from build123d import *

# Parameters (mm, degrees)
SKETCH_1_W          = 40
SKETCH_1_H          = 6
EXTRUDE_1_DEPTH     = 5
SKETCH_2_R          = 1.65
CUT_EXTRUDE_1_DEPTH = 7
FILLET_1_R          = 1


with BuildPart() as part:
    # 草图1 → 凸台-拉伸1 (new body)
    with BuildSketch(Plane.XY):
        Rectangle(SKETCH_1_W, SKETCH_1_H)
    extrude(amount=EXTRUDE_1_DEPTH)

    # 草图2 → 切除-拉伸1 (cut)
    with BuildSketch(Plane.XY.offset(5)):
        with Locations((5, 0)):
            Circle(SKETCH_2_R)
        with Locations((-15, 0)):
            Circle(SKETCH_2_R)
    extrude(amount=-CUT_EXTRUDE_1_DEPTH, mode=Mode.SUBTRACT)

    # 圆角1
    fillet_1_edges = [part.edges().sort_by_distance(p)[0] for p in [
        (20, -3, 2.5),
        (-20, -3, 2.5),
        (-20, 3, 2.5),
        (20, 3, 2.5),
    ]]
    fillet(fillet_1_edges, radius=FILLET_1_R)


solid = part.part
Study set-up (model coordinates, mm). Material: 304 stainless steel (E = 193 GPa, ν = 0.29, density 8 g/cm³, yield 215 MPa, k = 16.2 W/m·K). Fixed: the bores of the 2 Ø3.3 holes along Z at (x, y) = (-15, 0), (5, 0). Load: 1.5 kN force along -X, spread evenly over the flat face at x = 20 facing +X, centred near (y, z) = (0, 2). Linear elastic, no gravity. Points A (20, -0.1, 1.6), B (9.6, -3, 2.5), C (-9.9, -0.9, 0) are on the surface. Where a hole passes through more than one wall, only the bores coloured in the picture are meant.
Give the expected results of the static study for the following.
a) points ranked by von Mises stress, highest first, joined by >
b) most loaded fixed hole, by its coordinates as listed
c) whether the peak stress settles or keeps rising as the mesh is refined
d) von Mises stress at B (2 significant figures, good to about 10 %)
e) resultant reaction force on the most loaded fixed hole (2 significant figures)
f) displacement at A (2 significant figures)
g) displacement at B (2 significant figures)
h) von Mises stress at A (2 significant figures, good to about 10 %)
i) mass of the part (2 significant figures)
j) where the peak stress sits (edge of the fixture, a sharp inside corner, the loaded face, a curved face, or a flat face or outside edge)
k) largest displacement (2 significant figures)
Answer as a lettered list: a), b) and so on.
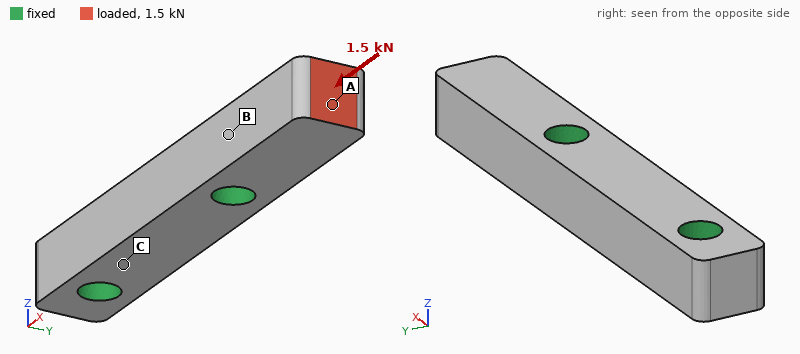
a) A > B > C
b) (5, 0)
c) keeps rising
d) 46 MPa
e) 1.5 kN
f) 4.0 µm
g) 1.0 µm
h) 61 MPa
i) 8.9 g
j) edge of the fixture
k) 4.1 µm
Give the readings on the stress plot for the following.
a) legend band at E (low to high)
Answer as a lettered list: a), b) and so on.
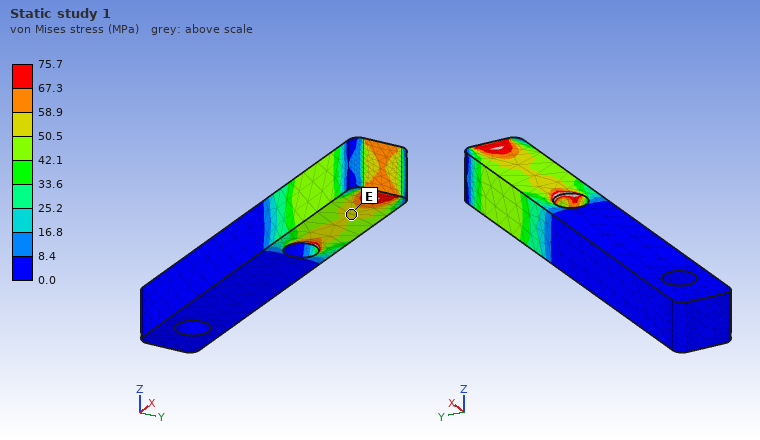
a) 50.5 to 58.9 MPa
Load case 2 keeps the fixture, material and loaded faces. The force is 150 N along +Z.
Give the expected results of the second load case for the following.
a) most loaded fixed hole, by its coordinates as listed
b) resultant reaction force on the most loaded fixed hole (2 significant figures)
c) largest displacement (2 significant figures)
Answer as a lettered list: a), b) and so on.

a) (5, 0)
b) 150 N
c) 13 µm
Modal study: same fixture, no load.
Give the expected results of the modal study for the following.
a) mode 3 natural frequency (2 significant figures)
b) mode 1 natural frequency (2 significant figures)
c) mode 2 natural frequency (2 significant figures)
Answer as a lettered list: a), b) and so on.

a) 50 kHz
b) 19 kHz
c) 19 kHz
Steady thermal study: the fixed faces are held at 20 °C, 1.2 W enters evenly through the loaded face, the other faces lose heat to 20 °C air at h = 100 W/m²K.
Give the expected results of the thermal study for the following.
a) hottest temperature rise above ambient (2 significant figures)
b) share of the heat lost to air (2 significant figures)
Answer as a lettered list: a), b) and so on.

a) 28 K
b) 33 %
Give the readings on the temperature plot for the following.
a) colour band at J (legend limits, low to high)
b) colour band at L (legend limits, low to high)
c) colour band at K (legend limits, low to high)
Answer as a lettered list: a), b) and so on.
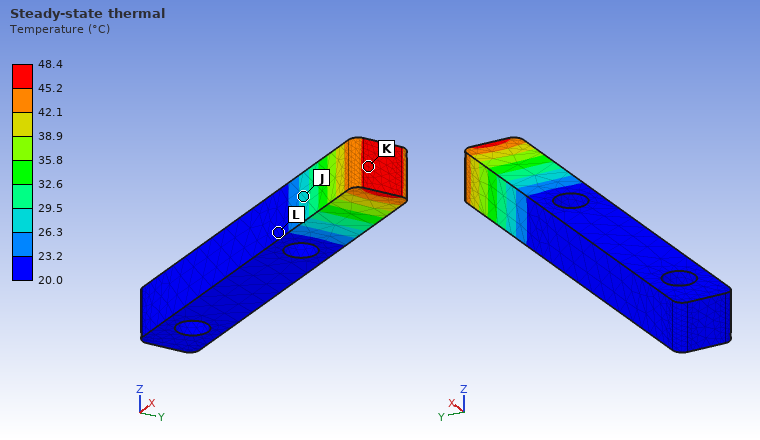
a) 26.3 to 29.5 °C
b) 20.0 to 23.2 °C
c) 45.2 to 48.4 °C
